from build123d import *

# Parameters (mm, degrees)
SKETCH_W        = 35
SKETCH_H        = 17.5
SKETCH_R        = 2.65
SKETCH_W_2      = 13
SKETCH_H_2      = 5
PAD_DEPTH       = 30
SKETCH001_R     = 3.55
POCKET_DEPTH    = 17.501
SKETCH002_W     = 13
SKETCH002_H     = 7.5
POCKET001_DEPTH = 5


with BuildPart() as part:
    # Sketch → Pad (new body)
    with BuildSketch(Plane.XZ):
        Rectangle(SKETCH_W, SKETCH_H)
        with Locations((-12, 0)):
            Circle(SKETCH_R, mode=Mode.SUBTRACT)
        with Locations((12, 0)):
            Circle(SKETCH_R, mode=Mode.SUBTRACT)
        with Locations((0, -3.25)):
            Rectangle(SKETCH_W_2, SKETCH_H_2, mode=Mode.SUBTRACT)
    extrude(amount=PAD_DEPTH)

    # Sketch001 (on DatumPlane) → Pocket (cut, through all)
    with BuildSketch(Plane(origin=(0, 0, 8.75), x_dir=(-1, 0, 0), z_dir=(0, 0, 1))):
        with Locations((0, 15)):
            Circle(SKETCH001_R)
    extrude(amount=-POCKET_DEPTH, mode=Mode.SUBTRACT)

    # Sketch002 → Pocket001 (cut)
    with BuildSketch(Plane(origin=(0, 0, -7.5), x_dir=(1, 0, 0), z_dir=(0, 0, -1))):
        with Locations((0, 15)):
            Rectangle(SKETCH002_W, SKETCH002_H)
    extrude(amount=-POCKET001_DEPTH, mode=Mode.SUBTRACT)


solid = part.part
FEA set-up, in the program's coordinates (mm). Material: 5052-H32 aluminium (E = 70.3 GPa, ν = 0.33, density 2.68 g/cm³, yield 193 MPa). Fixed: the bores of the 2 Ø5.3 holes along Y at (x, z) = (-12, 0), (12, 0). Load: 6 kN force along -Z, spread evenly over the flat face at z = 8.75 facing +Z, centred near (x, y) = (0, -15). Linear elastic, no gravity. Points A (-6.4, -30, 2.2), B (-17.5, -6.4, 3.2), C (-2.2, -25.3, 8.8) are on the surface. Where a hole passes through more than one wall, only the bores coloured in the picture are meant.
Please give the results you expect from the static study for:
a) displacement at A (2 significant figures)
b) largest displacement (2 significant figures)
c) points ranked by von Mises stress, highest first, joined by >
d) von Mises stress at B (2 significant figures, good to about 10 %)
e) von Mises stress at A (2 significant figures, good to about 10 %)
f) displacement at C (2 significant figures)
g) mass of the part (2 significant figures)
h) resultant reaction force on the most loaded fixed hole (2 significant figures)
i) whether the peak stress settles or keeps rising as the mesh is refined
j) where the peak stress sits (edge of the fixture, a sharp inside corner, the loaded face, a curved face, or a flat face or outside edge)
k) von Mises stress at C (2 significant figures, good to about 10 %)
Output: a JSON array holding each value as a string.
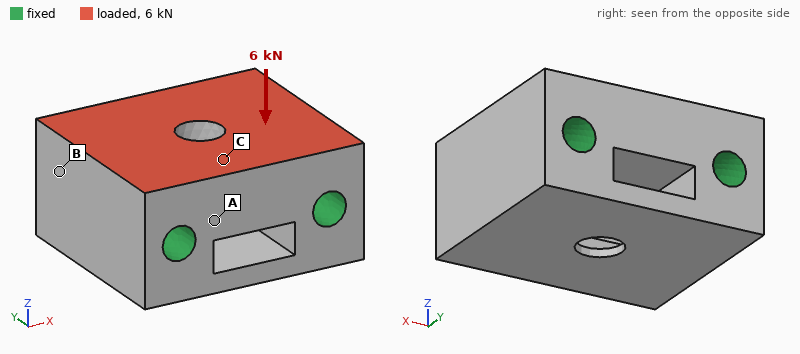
["1.1 µm", "2.4 µm", "A > C > B", "2.4 MPa", "11 MPa", "1.9 µm", "39 g", "3.1 kN", "keeps rising", "edge of the fixture", "7.3 MPa"]
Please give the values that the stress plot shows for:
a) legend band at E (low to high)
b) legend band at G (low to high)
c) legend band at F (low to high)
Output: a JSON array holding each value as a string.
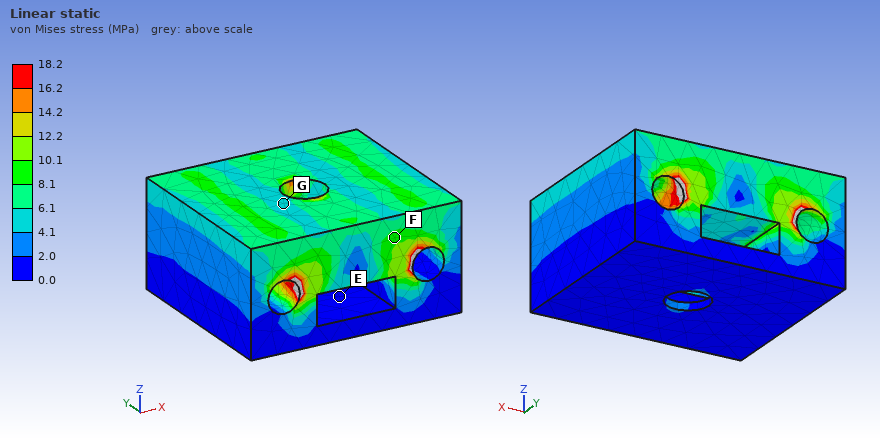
["0.0 to 2.0 MPa", "4.1 to 6.1 MPa", "8.1 to 10.1 MPa"]
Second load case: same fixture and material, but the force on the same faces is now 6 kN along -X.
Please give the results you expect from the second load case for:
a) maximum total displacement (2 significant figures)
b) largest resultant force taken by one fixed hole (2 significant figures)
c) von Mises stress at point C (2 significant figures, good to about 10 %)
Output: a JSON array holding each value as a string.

["3.8 µm", "3.3 kN", "11 MPa"]
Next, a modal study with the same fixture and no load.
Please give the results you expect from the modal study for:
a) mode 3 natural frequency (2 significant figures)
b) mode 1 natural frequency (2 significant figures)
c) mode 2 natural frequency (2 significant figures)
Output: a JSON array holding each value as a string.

["61 kHz", "50 kHz", "51 kHz"]
